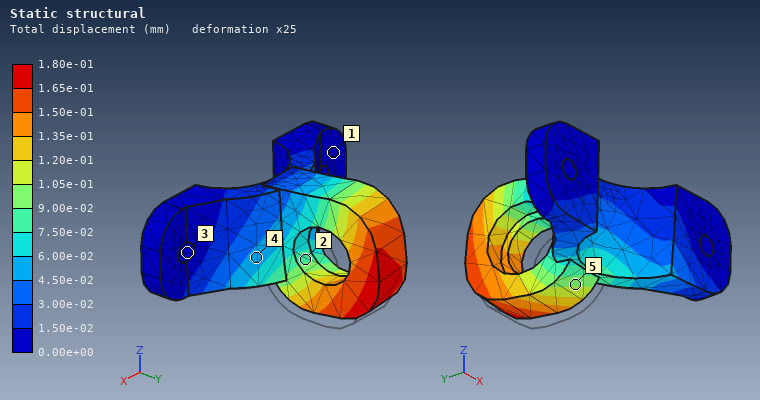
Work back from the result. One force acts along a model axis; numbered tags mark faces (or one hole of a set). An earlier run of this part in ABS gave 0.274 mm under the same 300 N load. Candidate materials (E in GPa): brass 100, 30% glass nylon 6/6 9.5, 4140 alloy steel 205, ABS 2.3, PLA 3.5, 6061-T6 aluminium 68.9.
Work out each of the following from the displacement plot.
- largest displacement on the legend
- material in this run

1.80e-01 mm
PLA
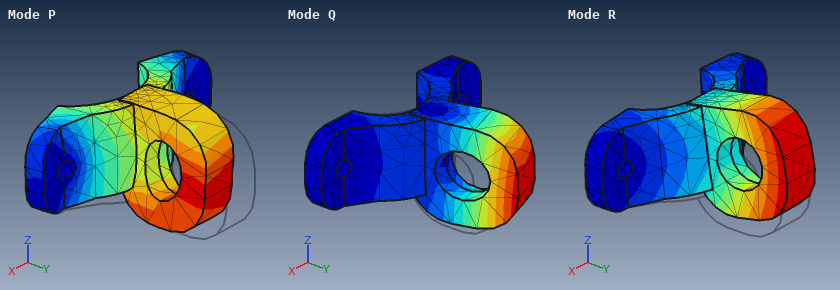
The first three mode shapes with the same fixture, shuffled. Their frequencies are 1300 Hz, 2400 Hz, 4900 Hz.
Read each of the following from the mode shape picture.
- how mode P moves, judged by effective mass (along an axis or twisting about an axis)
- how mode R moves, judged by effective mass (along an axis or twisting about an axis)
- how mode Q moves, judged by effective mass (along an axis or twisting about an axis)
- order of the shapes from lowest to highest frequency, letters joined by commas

along Y
along Z
along X
R, Q, P
